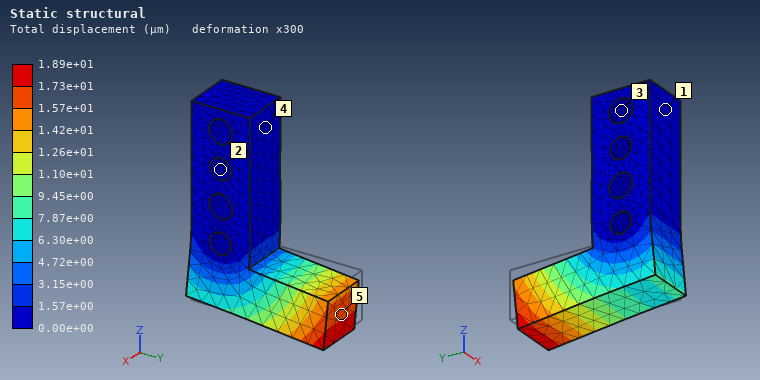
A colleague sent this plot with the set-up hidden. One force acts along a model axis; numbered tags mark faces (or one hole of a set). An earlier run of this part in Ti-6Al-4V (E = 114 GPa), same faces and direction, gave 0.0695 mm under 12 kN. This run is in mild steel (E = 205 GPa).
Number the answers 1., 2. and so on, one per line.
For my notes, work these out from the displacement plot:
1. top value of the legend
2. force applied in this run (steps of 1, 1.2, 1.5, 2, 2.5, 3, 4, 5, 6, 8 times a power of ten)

1. 1.89e+01 µm
2. 6 kN
